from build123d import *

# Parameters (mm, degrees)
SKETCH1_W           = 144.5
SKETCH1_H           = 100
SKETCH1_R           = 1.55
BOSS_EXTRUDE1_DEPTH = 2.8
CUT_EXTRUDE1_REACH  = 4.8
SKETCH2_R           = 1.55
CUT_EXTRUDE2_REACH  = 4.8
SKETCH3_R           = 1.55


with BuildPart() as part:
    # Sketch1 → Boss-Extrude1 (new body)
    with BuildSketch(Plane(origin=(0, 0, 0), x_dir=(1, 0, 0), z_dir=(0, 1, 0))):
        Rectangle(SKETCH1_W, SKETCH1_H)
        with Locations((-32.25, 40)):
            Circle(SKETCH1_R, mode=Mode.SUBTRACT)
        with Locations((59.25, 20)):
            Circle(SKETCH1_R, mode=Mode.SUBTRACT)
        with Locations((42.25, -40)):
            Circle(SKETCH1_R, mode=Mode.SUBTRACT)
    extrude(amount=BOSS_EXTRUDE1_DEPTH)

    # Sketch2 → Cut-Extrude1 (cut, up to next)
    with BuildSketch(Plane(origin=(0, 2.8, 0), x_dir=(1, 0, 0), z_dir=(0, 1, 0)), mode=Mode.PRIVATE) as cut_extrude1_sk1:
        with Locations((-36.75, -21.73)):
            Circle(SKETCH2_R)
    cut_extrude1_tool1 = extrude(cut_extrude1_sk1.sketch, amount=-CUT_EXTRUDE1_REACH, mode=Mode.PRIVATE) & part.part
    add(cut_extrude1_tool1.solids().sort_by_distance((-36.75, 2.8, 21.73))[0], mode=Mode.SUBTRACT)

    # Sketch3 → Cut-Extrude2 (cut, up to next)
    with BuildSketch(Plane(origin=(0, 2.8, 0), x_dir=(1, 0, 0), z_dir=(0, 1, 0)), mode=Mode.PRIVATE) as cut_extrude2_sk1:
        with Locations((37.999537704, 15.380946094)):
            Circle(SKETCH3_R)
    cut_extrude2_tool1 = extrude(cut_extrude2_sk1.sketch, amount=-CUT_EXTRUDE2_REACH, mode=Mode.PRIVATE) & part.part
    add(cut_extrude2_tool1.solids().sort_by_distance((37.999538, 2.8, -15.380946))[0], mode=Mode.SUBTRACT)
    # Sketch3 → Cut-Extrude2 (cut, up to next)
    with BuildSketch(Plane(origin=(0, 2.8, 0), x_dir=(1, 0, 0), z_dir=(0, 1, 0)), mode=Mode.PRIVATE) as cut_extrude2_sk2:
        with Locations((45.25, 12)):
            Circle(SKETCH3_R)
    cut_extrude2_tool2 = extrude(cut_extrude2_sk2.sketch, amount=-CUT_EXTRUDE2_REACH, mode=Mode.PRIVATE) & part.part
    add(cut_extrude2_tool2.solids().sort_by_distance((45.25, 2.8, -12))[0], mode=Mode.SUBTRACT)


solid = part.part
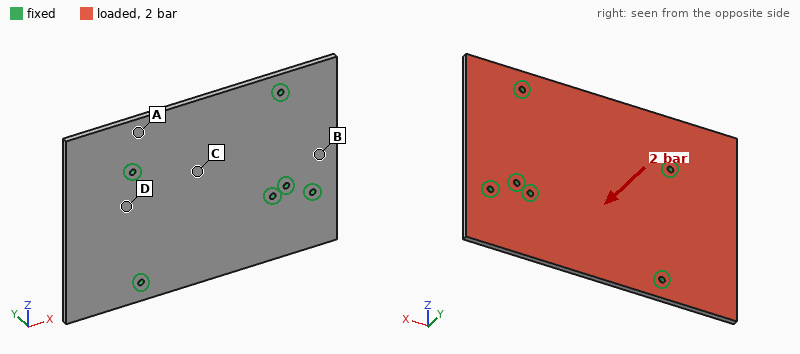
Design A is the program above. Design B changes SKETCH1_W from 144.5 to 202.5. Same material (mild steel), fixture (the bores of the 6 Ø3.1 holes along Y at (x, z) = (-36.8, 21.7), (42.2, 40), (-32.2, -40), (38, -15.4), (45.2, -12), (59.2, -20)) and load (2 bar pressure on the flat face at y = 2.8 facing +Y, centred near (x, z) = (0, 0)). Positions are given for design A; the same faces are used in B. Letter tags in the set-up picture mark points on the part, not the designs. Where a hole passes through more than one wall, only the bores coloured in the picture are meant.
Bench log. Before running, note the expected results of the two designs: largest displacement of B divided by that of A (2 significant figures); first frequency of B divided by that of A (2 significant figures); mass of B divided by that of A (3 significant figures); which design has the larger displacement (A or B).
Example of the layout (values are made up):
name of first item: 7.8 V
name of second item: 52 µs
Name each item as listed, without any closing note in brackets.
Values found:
largest displacement of B divided by that of A: 9.0
first frequency of B divided by that of A: 0.36
mass of B divided by that of A: 1.40
which design has the larger displacement: B
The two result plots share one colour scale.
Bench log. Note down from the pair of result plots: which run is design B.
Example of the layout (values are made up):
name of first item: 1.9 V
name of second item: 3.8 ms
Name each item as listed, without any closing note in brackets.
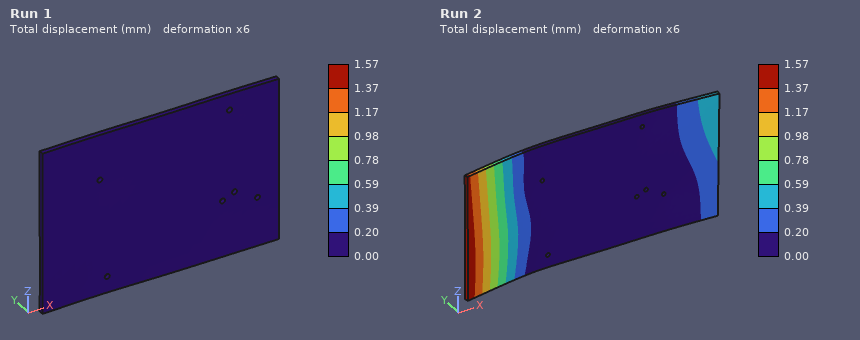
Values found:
which run is design B: Run 2
